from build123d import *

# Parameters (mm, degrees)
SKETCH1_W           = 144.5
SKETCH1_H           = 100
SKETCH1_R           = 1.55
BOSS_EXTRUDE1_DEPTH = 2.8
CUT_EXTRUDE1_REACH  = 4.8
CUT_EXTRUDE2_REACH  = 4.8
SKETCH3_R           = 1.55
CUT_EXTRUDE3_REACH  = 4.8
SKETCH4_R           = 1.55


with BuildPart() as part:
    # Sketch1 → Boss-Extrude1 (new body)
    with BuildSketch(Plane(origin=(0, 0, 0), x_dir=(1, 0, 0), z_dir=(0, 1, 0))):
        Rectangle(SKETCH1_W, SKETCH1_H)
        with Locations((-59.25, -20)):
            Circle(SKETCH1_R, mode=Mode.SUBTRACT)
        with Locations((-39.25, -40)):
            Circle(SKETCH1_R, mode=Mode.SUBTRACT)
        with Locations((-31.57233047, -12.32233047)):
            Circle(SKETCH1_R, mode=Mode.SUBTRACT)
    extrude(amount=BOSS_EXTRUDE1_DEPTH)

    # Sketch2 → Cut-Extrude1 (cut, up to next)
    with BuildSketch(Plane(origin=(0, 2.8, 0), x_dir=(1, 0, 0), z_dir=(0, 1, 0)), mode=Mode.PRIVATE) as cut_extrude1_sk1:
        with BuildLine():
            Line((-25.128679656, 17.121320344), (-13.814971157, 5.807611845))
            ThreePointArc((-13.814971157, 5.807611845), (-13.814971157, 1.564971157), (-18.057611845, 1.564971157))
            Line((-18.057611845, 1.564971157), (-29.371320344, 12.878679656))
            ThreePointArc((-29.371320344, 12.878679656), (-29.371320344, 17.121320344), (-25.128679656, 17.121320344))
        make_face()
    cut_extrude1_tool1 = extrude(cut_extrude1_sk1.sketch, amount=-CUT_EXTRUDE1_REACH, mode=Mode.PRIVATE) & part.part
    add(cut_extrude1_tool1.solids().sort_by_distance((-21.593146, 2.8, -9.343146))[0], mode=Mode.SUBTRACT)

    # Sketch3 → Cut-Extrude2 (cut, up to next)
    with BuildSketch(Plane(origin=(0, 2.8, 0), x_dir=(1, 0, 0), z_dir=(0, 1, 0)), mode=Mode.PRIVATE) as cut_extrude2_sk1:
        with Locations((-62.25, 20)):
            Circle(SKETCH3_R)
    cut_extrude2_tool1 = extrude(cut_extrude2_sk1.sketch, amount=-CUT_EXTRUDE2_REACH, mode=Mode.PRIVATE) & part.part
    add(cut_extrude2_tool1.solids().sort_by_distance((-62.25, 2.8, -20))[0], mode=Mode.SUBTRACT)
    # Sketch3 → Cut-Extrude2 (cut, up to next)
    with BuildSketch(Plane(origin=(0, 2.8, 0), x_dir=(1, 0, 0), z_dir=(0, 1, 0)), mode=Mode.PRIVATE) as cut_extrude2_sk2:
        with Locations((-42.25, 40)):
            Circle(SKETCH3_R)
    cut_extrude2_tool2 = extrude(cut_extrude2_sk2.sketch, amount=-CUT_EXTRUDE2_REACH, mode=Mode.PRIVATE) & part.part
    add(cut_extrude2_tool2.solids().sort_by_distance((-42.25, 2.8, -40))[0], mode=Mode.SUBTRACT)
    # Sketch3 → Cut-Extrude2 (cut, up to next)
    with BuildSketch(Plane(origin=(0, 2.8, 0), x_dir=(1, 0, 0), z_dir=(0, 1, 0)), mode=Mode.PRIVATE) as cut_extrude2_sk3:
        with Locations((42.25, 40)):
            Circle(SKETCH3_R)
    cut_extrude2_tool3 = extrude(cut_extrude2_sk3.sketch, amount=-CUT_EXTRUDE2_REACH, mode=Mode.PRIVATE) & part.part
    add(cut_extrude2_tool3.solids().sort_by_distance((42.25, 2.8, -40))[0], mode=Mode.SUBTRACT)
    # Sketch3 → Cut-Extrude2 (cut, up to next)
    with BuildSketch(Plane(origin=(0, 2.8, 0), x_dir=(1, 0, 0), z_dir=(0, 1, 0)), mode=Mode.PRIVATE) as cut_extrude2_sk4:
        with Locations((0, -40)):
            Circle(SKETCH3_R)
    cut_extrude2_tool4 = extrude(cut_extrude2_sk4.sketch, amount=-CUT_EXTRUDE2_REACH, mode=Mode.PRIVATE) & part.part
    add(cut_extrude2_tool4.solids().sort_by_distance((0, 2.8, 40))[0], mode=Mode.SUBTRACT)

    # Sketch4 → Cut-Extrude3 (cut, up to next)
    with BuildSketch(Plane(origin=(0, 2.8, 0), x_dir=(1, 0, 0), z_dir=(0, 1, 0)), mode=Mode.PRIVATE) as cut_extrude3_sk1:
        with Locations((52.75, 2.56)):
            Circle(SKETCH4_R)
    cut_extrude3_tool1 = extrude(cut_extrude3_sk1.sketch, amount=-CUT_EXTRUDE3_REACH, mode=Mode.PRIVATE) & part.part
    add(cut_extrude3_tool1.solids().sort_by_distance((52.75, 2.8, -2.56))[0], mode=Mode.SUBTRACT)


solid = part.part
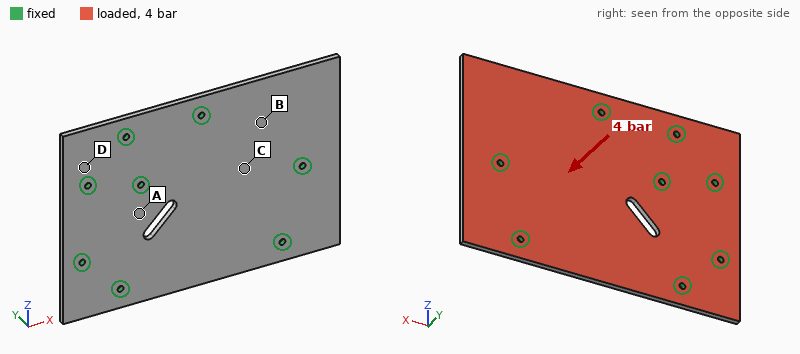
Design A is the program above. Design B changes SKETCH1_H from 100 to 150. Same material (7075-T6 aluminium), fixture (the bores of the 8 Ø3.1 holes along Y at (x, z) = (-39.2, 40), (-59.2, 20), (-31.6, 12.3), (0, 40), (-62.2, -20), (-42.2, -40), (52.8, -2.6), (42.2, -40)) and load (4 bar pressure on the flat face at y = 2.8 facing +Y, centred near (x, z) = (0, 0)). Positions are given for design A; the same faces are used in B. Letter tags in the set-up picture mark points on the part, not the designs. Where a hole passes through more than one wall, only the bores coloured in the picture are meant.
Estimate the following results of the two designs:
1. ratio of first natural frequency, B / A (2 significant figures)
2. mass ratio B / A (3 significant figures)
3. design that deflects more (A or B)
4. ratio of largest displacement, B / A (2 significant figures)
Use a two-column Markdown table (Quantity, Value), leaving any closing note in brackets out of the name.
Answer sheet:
| Quantity | Value |
|---|---|
| ratio of first natural frequency, B / A | 0.59 |
| mass ratio B / A | 1.51 |
| design that deflects more | B |
| ratio of largest displacement, B / A | 3.2 |
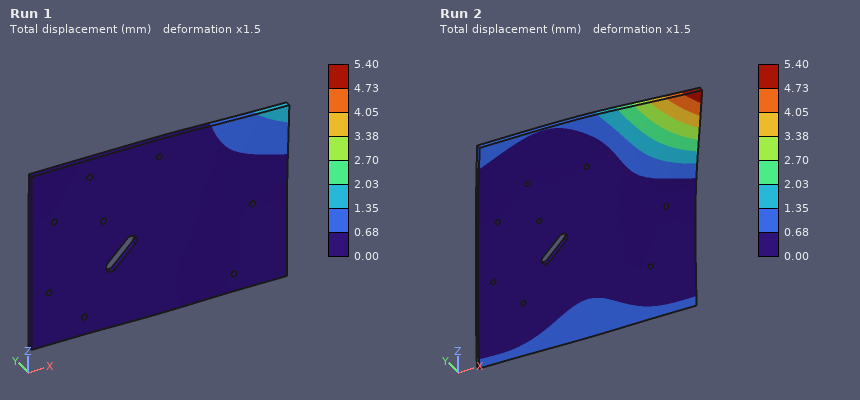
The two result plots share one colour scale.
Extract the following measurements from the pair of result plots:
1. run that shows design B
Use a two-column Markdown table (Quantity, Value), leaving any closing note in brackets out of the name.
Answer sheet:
| Quantity | Value |
|---|---|
| run that shows design B | Run 2 |
